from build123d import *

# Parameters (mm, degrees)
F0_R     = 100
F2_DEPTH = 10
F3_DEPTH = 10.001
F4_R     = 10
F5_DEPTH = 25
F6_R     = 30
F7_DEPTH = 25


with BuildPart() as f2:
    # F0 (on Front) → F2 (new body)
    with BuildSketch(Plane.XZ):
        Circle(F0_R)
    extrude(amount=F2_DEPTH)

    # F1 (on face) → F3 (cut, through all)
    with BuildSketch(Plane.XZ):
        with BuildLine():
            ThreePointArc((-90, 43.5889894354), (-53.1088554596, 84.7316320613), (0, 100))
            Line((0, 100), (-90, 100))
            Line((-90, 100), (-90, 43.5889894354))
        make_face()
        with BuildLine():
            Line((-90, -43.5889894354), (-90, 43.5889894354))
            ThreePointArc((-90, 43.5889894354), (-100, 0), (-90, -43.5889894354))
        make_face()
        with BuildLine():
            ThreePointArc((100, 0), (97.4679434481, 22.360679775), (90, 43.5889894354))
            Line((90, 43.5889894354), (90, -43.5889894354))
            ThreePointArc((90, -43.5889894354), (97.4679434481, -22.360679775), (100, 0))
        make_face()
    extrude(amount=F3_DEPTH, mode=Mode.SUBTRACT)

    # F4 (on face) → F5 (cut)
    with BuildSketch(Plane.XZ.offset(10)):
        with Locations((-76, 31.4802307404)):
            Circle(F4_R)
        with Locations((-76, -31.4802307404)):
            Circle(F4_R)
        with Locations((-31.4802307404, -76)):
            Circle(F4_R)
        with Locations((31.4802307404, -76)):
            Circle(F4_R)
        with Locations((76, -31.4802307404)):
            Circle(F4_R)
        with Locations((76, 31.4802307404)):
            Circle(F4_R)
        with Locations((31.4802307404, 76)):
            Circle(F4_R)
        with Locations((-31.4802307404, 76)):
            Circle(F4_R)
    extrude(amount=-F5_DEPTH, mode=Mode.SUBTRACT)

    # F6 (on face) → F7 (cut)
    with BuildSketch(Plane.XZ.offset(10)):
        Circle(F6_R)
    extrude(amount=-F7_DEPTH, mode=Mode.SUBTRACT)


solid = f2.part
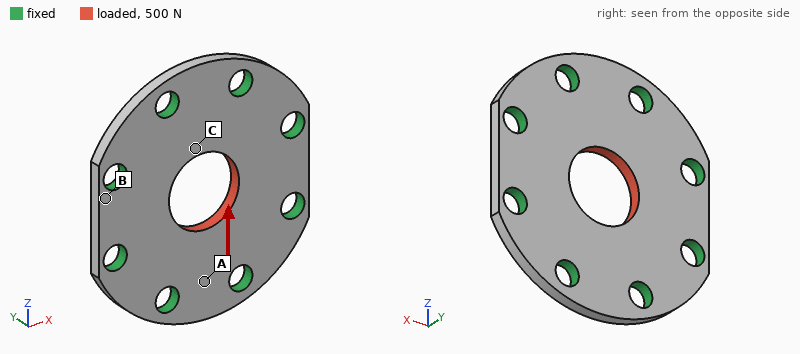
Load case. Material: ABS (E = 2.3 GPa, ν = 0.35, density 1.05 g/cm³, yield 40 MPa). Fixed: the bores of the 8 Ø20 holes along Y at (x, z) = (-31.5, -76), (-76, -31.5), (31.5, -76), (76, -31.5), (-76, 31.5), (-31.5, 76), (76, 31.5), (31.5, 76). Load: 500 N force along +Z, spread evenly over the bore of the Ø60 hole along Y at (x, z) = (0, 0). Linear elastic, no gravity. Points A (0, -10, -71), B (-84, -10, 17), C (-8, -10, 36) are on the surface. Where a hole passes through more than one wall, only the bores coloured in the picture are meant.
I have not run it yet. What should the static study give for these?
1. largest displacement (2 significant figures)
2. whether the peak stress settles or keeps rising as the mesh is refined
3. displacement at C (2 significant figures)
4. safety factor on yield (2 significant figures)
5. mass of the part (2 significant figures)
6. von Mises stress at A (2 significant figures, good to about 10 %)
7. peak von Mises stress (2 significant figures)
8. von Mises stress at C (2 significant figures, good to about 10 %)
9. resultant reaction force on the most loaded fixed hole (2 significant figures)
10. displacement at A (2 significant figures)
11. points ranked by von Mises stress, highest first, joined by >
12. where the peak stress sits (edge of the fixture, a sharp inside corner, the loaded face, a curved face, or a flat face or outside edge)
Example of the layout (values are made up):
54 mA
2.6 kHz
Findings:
5.6 µm
settles
4.5 µm
87
260 g
0.089 MPa
0.46 MPa
0.25 MPa
97 N
2.0 µm
C > A > B
the loaded face
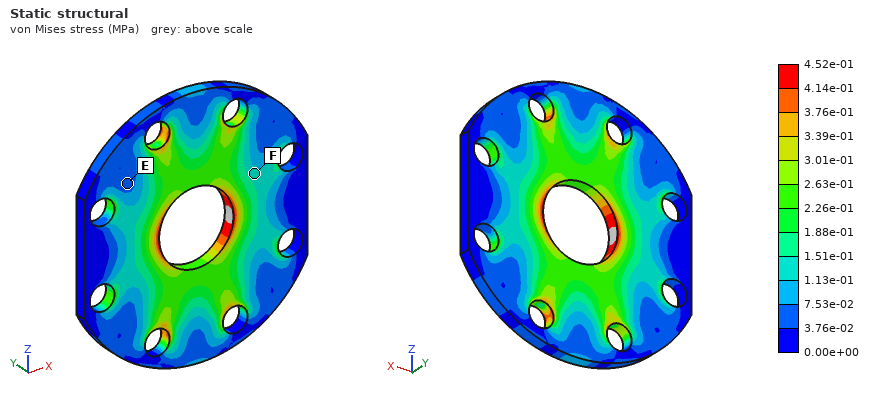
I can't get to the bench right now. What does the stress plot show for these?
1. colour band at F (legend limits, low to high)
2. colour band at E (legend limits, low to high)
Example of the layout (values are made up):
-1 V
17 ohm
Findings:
1.13e-01 to 1.51e-01 MPa
3.76e-02 to 7.53e-02 MPa
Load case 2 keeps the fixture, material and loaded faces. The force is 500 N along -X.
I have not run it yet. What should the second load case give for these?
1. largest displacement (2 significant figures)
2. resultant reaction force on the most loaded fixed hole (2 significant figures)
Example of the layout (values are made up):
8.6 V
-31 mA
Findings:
5.6 µm
98 N
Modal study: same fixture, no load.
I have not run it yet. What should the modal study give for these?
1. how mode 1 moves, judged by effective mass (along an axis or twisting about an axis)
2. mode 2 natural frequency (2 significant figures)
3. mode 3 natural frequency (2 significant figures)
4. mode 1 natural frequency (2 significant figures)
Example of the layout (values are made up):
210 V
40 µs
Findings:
along Y
2000 Hz
2100 Hz
1500 Hz
